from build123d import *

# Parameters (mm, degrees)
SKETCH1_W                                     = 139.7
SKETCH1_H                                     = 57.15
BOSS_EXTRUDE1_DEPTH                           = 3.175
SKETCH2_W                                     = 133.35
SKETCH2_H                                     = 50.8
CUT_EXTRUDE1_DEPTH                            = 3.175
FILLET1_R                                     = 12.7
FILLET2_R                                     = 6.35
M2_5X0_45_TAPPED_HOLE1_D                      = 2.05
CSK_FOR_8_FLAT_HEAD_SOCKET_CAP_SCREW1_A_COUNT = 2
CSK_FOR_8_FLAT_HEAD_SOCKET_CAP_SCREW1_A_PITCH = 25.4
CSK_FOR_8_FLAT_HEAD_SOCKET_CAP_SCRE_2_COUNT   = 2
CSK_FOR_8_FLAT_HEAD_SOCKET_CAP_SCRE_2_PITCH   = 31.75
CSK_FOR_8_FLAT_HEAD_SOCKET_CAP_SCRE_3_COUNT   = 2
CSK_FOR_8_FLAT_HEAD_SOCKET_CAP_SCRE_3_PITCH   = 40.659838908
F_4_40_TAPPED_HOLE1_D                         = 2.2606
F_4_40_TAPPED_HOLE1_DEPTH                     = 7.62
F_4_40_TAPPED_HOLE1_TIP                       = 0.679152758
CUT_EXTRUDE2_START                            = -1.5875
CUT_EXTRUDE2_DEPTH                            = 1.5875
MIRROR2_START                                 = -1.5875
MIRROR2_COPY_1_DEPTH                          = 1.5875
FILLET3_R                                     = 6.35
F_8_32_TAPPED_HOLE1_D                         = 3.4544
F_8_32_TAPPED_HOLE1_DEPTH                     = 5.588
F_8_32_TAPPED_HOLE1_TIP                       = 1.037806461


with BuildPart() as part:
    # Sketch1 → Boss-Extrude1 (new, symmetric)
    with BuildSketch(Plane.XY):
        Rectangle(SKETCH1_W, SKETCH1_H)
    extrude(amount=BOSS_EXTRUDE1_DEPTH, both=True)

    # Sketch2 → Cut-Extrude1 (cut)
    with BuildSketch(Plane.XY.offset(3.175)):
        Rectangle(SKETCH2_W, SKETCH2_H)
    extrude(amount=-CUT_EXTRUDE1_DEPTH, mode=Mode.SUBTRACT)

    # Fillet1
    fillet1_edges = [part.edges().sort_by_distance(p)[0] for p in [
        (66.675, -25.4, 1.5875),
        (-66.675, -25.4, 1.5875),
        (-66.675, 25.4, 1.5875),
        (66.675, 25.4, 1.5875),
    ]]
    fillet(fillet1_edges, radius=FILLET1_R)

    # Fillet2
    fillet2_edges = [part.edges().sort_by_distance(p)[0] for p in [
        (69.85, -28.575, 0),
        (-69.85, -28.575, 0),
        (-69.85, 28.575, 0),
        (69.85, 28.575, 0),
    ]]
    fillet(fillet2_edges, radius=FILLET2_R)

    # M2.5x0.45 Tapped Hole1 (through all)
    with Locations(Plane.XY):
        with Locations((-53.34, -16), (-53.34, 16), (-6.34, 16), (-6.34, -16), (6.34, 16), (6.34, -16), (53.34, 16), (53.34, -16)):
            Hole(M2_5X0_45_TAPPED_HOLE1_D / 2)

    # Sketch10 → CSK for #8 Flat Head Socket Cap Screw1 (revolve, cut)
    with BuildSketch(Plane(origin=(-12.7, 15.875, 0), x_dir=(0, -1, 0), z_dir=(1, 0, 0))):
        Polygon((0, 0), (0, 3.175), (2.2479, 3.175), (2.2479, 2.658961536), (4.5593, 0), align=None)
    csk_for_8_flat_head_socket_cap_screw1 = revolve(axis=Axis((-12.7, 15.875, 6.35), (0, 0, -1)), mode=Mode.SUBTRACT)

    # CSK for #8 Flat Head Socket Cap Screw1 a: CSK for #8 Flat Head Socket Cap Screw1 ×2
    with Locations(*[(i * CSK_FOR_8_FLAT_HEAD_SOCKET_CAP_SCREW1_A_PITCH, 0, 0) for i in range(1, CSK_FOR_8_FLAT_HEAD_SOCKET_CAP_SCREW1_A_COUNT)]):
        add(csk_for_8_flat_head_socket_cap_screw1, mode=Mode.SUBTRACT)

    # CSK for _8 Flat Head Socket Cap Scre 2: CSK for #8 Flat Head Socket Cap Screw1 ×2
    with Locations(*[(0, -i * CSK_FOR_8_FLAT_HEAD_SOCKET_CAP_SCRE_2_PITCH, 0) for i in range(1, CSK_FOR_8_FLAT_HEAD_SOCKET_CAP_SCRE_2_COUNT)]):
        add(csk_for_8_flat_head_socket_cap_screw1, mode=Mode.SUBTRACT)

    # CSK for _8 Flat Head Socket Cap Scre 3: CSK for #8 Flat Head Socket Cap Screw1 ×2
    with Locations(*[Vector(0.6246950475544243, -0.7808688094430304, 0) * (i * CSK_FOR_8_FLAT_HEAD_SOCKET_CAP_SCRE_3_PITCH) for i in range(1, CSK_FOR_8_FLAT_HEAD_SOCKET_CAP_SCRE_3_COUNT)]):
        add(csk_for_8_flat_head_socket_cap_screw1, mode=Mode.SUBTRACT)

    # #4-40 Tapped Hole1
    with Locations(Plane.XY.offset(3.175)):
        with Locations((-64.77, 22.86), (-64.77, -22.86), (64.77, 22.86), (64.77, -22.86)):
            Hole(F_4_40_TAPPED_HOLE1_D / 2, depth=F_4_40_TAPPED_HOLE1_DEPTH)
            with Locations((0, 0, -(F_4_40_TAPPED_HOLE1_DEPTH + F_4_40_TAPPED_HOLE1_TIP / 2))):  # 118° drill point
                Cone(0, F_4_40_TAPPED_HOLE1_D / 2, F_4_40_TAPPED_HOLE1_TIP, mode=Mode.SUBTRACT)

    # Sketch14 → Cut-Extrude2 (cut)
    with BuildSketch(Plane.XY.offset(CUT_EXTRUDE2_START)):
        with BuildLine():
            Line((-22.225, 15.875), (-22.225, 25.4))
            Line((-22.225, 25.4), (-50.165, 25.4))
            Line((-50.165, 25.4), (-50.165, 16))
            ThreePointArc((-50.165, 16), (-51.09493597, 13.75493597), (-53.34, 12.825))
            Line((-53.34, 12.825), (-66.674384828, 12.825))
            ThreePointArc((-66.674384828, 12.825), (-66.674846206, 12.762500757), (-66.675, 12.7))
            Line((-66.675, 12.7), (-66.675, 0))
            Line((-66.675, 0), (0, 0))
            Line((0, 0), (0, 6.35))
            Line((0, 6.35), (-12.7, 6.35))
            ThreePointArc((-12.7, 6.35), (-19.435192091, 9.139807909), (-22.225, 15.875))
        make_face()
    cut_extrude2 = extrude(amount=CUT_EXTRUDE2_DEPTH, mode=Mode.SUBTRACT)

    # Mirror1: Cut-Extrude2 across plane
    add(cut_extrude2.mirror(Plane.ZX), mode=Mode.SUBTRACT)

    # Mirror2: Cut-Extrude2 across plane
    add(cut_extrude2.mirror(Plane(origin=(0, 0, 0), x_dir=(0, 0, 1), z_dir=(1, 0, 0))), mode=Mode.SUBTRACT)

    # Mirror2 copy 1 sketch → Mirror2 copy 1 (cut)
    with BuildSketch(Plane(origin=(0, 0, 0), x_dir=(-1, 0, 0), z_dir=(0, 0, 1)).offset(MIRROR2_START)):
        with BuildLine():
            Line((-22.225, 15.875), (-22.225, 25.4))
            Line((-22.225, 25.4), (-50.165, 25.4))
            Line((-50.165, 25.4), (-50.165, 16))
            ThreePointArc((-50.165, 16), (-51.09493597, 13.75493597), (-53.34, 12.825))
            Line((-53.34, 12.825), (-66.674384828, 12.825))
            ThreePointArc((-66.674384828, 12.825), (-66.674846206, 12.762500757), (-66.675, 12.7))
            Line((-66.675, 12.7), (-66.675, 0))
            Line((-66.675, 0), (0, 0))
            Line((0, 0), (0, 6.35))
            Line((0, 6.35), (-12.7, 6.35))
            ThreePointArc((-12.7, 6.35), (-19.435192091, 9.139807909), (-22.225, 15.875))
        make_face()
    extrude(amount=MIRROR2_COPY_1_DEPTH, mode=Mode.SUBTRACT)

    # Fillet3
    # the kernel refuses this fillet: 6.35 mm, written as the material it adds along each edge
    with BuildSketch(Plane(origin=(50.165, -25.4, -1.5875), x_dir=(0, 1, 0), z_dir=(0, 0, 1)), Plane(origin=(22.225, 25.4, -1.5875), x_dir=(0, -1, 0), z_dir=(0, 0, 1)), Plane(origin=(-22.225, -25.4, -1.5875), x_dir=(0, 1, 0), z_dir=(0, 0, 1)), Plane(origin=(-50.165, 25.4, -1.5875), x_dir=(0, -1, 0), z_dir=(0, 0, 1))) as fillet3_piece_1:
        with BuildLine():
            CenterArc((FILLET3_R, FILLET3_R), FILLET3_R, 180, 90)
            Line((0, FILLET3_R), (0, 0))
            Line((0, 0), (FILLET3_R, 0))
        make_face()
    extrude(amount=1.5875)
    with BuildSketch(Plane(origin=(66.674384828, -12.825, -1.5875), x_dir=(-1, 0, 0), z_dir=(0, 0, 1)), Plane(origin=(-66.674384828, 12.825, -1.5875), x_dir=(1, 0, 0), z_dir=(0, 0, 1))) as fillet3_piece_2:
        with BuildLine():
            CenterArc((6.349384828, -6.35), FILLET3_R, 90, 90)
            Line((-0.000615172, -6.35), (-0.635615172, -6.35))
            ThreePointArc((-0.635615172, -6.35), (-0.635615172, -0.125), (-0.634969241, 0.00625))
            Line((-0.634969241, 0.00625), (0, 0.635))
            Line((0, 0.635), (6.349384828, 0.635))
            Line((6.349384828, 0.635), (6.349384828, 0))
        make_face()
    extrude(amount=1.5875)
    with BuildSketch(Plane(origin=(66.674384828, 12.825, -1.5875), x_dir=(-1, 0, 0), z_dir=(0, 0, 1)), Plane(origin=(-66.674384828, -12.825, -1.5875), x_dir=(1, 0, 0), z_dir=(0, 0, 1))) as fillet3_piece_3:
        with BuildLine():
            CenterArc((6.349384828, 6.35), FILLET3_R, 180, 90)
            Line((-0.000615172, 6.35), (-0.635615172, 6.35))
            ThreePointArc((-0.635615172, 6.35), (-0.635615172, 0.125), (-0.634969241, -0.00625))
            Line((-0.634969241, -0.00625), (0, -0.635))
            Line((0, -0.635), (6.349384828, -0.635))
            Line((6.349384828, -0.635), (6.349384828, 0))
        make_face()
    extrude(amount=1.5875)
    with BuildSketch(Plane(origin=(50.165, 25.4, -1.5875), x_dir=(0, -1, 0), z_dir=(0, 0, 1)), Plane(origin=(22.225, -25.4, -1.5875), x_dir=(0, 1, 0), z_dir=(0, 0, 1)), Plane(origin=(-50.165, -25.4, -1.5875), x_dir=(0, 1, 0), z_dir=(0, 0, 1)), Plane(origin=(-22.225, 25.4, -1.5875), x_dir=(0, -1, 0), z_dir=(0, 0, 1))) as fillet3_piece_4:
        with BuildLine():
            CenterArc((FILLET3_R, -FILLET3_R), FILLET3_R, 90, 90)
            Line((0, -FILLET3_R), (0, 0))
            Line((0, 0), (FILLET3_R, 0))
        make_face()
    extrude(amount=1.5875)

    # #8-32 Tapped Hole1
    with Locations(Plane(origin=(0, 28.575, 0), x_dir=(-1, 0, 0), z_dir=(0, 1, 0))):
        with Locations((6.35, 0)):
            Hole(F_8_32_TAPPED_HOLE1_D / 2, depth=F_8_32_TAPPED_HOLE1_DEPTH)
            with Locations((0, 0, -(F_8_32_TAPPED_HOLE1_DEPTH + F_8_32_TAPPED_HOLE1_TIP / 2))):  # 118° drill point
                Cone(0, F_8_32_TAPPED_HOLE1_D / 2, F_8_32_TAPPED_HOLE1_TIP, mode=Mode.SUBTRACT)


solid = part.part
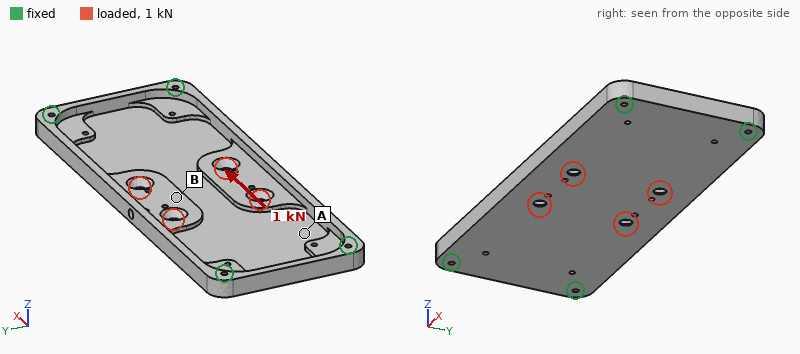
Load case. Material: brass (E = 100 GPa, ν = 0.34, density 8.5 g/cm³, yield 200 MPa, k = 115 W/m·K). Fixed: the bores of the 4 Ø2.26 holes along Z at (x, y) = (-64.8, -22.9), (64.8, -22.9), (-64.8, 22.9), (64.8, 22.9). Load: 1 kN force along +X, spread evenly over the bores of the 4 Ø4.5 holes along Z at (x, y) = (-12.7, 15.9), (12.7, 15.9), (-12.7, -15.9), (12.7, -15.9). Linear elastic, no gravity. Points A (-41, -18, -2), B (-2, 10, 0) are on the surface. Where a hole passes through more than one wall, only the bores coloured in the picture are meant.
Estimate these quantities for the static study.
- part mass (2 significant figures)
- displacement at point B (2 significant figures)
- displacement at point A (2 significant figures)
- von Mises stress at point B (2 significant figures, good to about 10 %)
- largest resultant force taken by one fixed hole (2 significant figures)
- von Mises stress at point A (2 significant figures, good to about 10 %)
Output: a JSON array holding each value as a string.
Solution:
["190 g", "2.3 µm", "1.4 µm", "2.6 MPa", "250 N", "5.5 MPa"]
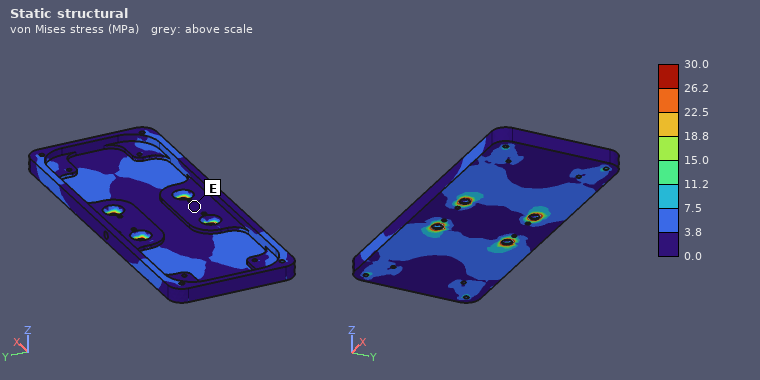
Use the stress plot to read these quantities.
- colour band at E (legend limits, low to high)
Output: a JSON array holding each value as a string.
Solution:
["0.0 to 3.8 MPa"]
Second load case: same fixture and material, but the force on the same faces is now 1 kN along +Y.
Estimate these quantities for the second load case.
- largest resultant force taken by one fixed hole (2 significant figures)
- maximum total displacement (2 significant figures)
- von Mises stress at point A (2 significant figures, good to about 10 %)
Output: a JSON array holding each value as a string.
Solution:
["400 N", "18 µm", "11 MPa"]
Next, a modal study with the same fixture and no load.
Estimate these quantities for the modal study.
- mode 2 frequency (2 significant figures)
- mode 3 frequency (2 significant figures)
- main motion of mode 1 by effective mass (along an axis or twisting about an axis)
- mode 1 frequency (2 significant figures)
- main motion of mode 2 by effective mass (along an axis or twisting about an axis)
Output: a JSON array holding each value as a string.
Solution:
["1300 Hz", "2300 Hz", "along Z", "870 Hz", "twisting about X"]
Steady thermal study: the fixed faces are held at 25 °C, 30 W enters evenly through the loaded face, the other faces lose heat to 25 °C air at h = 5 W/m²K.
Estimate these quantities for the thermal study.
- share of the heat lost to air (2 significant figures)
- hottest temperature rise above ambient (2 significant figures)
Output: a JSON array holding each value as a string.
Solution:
["9.2 %", "59 K"]
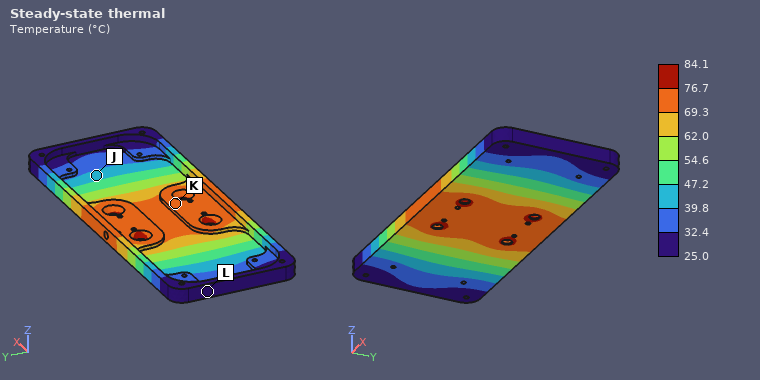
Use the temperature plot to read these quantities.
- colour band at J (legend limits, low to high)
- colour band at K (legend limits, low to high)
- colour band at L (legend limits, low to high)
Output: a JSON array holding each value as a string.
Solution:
["39.8 to 47.2 °C", "69.3 to 76.7 °C", "25.0 to 32.4 °C"]
